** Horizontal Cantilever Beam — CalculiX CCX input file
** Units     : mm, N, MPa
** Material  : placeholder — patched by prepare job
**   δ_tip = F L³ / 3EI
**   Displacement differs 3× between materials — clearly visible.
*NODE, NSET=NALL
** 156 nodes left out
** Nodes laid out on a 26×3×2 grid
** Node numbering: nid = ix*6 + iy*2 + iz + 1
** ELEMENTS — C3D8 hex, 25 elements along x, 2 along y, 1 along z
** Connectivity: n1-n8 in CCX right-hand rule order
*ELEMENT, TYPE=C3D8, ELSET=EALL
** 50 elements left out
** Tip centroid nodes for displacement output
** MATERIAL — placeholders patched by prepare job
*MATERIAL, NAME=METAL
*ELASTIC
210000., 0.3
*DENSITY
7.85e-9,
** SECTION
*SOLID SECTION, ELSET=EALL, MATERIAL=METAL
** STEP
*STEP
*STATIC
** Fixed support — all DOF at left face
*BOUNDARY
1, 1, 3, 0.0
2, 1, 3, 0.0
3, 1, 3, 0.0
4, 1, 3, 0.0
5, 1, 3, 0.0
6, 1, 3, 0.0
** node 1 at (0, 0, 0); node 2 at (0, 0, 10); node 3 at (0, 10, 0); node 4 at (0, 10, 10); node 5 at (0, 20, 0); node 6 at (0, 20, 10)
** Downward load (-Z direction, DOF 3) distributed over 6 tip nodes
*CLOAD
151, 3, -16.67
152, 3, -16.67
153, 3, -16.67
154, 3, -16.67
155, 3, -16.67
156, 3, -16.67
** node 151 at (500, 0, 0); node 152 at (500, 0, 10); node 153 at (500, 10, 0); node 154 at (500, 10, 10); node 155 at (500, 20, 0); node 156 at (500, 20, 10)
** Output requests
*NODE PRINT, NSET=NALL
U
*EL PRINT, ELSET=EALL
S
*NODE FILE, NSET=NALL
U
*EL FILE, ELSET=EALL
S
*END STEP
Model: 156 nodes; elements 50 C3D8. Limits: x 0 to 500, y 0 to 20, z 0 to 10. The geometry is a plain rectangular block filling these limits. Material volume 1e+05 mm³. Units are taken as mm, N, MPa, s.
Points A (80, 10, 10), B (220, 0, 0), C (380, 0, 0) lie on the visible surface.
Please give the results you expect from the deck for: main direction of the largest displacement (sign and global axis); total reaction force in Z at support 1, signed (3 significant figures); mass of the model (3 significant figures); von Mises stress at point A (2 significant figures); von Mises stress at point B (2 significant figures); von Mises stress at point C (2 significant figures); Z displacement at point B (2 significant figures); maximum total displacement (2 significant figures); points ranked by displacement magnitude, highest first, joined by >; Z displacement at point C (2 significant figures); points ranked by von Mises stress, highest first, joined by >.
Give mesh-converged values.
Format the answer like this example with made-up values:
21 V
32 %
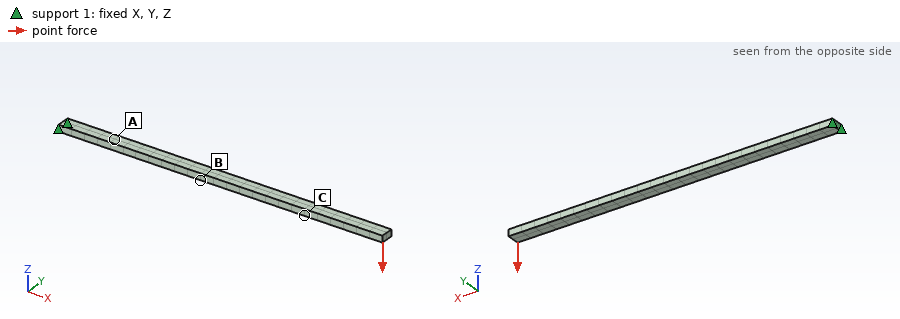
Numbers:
-Z
100 N
0.785 kg
130 MPa
84 MPa
36 MPa
-2.9 mm
12 mm
C > B > A
-7.7 mm
A > B > C
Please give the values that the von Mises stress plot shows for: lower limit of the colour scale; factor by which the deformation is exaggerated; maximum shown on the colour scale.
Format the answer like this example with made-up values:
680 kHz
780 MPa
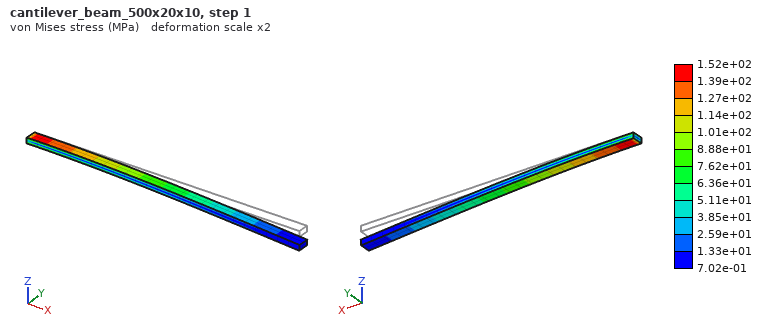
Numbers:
7.02e-01 MPa
2
1.52e+02 MPa
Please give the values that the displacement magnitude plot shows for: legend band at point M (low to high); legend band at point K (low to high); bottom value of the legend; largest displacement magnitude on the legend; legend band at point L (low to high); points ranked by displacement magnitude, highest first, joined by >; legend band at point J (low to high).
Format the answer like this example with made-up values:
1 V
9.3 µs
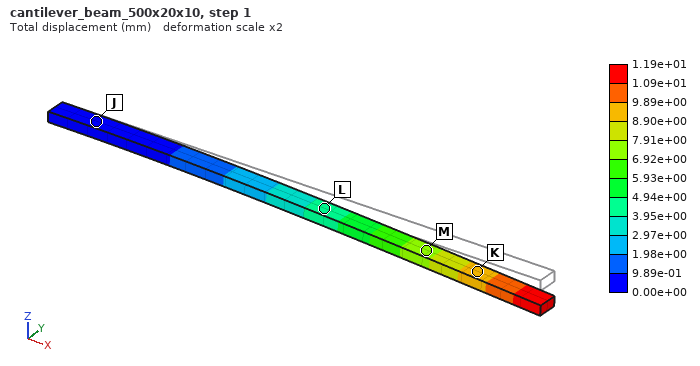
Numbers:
6.92e+00 to 7.91e+00 mm
8.90e+00 to 9.89e+00 mm
0.00e+00 mm
1.19e+01 mm
3.95e+00 to 4.94e+00 mm
K > M > L > J
0.00e+00 to 9.89e-01 mm
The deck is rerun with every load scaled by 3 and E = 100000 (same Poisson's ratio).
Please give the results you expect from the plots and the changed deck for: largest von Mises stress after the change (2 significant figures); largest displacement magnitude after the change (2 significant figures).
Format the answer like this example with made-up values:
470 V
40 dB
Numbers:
460 MPa
75 mm
